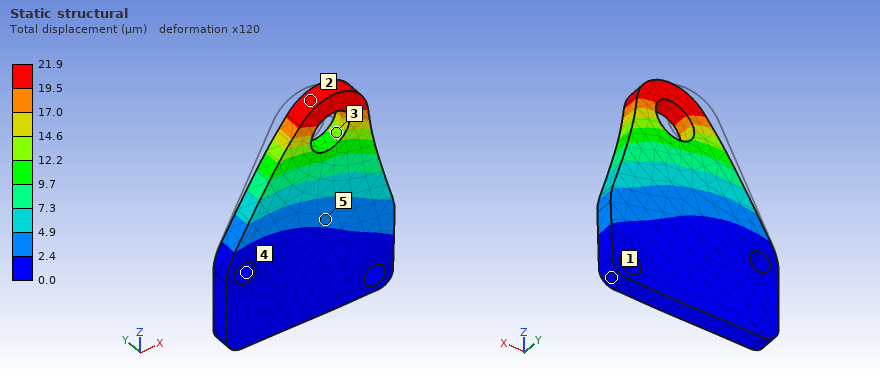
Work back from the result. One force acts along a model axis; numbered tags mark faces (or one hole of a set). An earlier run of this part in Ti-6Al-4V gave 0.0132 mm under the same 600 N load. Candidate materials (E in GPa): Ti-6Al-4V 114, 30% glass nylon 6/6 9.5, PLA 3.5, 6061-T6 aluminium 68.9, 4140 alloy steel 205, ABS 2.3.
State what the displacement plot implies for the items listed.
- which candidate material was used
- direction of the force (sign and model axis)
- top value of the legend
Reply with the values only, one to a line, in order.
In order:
6061-T6 aluminium
+X
21.9 µm
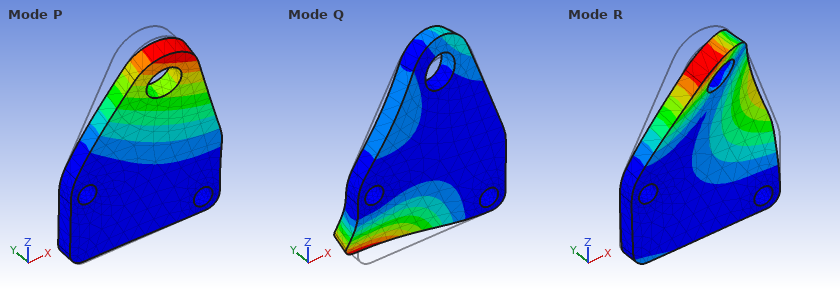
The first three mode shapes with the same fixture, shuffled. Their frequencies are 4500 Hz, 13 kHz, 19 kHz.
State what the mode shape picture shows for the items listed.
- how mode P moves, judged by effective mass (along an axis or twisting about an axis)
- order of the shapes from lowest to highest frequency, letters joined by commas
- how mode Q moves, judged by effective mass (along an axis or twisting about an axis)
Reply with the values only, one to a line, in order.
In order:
along Y
P, R, Q
along Y
